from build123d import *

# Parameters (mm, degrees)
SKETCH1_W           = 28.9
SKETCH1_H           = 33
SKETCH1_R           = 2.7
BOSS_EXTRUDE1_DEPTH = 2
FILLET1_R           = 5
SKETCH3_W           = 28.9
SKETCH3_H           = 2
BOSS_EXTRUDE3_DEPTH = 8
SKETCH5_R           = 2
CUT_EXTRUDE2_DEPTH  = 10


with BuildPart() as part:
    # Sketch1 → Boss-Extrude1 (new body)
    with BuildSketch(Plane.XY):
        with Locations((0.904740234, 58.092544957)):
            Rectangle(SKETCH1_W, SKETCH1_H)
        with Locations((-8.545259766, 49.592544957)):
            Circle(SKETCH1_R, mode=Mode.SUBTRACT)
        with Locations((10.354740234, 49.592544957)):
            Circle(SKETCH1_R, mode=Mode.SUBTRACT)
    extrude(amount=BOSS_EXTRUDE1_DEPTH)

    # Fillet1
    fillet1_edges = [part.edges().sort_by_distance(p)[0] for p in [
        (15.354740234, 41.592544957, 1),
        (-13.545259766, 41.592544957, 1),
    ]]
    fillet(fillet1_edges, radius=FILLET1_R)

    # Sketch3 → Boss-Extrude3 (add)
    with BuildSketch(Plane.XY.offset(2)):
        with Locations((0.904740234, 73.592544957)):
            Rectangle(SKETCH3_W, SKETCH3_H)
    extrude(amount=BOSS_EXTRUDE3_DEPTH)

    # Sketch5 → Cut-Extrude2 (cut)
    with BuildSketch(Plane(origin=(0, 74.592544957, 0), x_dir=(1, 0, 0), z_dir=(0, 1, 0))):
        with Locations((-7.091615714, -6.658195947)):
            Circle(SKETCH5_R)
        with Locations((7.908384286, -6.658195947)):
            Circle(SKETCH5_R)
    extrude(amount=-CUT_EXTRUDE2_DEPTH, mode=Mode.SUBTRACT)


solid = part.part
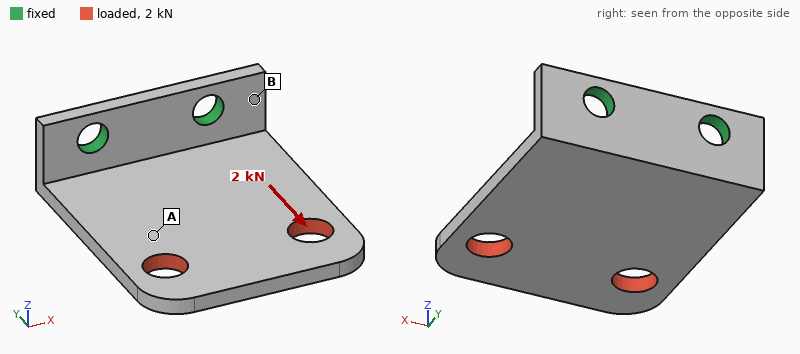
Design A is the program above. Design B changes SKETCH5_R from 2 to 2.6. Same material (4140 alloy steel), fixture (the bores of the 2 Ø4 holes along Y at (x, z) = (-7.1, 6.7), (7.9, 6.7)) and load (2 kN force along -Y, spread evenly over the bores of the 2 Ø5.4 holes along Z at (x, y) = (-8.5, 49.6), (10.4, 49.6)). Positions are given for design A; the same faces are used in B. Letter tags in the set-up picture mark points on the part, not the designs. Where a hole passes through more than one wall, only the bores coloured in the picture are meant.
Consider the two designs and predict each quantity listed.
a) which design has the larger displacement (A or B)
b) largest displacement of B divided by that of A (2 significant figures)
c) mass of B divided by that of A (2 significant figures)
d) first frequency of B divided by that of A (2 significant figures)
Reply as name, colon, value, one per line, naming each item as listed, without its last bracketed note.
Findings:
which design has the larger displacement: A
largest displacement of B divided by that of A: 0.72
mass of B divided by that of A: 0.98
first frequency of B divided by that of A: 1.0
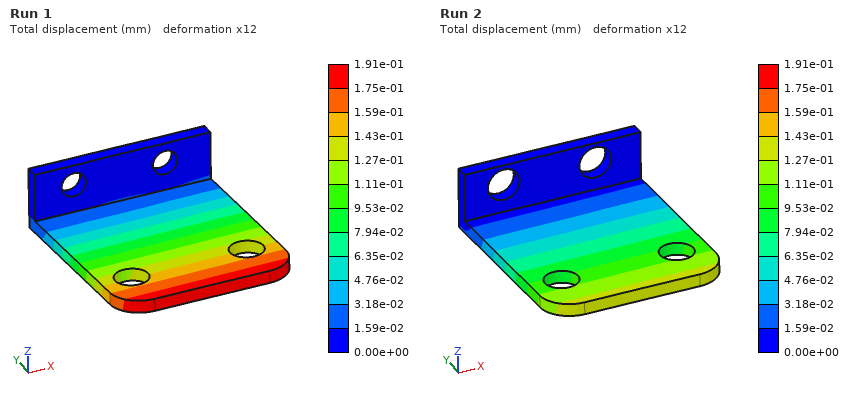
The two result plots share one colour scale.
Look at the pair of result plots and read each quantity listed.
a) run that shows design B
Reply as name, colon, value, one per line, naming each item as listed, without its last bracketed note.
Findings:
run that shows design B: Run 2
